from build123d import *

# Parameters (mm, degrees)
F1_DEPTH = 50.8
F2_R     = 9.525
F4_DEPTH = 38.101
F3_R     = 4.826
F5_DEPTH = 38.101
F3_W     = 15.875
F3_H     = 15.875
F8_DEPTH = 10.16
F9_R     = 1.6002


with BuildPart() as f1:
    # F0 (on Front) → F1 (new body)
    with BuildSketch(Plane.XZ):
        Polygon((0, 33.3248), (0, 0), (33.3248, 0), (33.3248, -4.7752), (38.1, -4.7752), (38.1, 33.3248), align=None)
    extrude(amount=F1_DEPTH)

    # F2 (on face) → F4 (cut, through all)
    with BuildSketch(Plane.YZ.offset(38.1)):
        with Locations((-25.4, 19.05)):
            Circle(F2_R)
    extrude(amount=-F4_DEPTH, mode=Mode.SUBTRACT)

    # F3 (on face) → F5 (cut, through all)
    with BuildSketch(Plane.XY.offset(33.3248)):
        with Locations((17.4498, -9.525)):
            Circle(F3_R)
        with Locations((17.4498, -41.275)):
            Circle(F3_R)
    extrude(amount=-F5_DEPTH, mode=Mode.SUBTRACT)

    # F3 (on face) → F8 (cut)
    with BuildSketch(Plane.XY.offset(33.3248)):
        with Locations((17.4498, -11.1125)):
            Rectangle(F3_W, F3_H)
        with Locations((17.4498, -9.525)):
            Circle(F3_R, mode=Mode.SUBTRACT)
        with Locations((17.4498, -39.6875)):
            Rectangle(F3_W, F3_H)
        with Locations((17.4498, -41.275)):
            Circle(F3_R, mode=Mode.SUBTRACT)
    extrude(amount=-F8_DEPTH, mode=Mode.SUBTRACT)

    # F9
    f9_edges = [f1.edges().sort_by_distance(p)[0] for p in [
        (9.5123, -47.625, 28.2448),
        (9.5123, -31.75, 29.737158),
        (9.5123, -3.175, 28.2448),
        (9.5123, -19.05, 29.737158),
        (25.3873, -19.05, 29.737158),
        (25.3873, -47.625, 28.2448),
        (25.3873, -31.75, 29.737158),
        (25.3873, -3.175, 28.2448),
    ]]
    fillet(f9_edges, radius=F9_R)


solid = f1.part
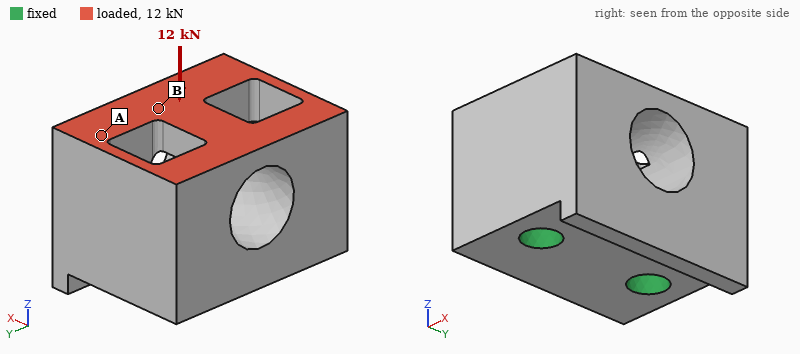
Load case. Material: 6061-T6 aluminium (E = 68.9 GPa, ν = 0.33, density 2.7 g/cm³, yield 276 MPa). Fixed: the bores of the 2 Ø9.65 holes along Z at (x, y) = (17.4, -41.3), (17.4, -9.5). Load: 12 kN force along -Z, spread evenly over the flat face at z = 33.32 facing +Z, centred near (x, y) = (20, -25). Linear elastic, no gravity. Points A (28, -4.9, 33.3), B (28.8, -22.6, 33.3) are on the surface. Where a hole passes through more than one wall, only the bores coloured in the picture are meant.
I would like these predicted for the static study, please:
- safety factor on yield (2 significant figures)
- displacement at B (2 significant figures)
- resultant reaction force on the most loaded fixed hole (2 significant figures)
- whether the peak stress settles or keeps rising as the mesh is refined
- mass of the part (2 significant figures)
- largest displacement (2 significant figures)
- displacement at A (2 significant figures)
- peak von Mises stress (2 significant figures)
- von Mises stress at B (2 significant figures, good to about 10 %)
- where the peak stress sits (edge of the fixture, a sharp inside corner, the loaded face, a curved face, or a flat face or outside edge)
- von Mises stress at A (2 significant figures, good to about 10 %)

1.6
15 µm
6.1 kN
settles
130 g
23 µm
5.8 µm
170 MPa
38 MPa
a curved face
12 MPa
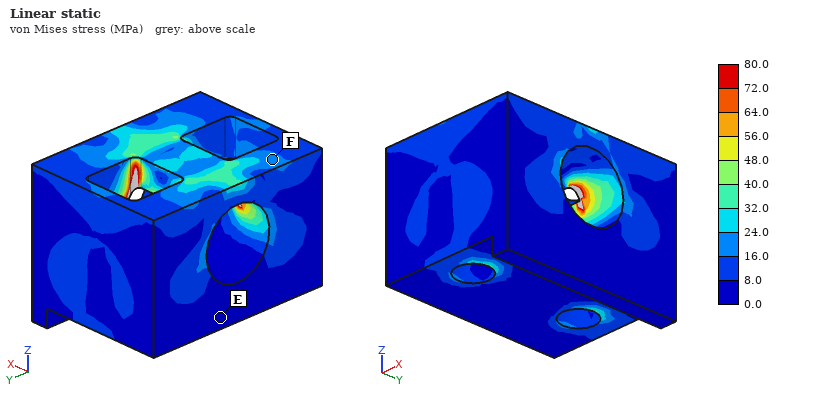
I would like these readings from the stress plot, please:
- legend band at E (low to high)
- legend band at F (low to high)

0.0 to 8.0 MPa
16.0 to 24.0 MPa
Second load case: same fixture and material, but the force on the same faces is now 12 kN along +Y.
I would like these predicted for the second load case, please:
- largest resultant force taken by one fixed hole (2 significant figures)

7.0 kN
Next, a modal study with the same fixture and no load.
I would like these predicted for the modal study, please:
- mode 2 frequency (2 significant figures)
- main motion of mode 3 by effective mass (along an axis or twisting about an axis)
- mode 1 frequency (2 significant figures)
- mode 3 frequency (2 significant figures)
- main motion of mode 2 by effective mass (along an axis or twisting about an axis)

21 kHz
twisting about Z
19 kHz
24 kHz
along Y
